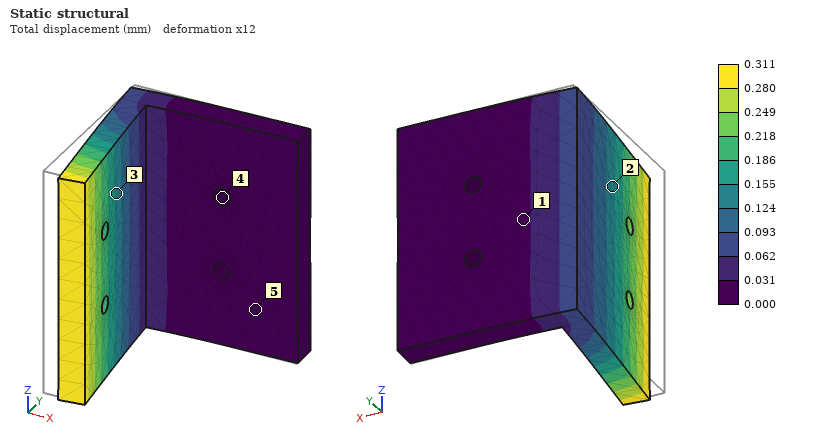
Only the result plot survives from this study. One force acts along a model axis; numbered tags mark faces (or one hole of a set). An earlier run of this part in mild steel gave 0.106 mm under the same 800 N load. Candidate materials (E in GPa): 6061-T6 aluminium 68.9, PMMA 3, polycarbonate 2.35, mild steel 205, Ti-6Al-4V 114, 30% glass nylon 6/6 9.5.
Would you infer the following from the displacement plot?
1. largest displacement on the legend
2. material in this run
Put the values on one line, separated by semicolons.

0.311 mm; 6061-T6 aluminium
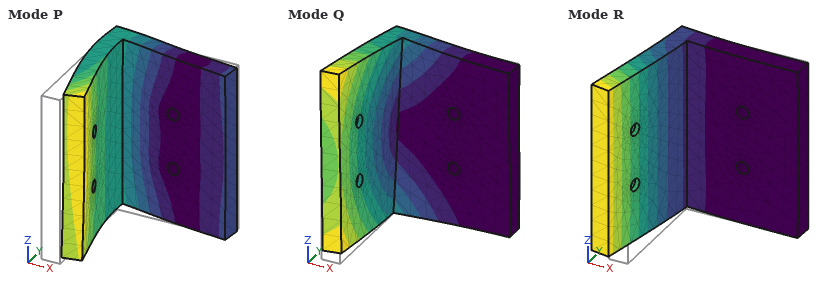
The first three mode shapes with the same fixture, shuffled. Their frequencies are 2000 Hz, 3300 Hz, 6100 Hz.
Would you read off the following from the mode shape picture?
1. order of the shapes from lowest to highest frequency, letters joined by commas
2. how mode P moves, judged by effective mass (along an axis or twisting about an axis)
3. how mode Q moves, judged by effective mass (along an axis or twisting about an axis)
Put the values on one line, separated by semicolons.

R, Q, P; along Y; along Z
